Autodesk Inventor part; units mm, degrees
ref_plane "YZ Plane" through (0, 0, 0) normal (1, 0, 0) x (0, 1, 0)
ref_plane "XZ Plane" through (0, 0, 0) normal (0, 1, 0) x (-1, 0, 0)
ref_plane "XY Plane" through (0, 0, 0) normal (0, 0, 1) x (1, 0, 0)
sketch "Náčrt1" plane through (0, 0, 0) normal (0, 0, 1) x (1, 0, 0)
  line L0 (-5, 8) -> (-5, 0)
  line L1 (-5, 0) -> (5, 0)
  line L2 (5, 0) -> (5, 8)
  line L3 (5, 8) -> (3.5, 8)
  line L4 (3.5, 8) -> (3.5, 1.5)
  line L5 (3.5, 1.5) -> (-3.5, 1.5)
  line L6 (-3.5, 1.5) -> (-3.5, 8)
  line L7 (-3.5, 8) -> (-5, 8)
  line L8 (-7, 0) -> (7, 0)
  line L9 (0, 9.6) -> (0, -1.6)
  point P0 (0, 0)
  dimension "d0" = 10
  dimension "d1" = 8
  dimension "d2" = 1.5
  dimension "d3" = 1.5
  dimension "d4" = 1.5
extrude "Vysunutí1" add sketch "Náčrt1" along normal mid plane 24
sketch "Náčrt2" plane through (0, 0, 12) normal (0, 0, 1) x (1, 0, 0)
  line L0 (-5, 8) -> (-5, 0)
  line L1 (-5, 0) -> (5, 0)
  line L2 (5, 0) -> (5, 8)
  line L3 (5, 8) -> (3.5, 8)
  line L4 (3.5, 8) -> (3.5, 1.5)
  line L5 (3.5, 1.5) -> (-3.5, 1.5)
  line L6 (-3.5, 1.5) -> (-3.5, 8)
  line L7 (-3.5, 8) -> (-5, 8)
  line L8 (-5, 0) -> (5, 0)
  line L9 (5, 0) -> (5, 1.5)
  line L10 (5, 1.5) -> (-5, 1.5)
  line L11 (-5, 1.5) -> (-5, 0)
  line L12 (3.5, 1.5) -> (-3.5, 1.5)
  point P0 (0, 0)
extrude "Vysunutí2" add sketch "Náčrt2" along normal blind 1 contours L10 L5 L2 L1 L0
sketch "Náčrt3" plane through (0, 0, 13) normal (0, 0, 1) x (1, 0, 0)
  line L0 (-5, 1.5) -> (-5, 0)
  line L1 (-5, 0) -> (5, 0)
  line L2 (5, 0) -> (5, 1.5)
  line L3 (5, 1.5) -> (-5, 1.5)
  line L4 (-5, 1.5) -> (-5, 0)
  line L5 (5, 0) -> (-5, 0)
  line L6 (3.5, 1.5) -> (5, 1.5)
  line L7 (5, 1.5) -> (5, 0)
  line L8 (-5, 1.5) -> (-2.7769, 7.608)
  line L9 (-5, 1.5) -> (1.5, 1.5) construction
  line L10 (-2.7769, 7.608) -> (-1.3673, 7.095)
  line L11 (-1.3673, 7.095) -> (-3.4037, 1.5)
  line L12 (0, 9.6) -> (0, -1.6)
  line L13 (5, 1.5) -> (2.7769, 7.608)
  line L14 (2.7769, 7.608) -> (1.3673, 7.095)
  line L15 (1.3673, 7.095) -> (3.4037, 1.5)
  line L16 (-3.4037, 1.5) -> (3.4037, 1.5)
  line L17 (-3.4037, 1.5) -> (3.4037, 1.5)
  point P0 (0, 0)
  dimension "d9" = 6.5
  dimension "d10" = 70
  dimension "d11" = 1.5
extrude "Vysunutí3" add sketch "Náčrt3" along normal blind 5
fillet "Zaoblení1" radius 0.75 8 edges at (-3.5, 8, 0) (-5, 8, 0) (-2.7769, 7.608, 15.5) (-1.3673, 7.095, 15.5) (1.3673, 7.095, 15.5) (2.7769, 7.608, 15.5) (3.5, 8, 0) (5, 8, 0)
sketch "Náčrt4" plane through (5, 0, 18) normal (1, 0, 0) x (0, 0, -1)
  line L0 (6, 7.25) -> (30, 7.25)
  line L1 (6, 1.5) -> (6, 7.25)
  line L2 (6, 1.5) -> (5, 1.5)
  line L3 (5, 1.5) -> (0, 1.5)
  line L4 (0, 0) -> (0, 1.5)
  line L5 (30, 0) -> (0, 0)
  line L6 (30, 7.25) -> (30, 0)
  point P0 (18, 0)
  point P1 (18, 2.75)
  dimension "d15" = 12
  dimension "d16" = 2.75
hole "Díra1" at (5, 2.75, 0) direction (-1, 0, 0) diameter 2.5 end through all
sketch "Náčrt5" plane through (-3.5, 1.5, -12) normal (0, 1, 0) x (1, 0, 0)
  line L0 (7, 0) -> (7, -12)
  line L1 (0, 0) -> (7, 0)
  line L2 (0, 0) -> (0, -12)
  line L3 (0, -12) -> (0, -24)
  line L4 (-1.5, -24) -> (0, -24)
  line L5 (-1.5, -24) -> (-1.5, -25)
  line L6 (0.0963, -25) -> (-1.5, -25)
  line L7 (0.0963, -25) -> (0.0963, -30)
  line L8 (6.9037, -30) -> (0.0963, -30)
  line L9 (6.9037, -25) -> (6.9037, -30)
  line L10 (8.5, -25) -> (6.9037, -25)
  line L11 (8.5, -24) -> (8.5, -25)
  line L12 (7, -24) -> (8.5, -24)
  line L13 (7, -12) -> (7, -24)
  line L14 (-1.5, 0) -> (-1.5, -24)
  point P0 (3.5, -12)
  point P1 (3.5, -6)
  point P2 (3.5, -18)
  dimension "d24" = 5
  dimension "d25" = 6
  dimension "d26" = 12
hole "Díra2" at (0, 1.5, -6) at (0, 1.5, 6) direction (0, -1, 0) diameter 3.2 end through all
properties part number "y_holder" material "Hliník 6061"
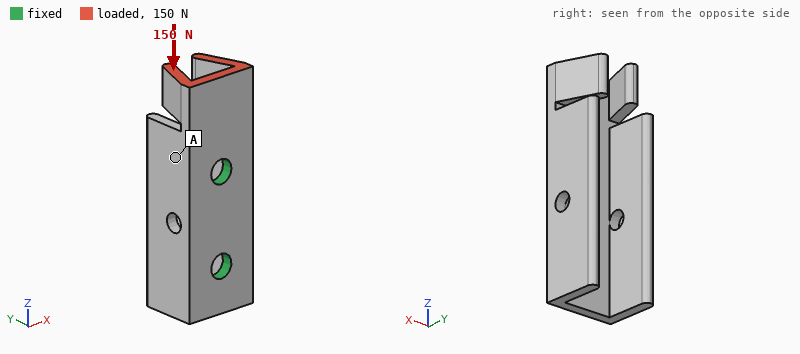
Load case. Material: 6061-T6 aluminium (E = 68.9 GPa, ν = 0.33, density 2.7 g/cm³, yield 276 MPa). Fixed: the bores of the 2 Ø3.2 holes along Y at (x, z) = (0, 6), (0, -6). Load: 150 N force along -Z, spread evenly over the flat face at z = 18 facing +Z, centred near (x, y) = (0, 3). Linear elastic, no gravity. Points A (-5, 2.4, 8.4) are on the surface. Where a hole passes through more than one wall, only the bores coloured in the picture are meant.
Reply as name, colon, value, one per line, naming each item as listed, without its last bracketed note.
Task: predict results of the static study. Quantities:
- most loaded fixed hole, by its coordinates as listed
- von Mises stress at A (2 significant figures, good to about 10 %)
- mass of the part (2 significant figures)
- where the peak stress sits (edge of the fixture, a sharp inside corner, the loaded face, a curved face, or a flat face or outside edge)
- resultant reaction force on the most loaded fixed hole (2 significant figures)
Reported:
most loaded fixed hole, by its coordinates as listed: (0, 6)
von Mises stress at A: 12 MPa
mass of the part: 2.6 g
where the peak stress sits: a flat face or outside edge
resultant reaction force on the most loaded fixed hole: 110 N
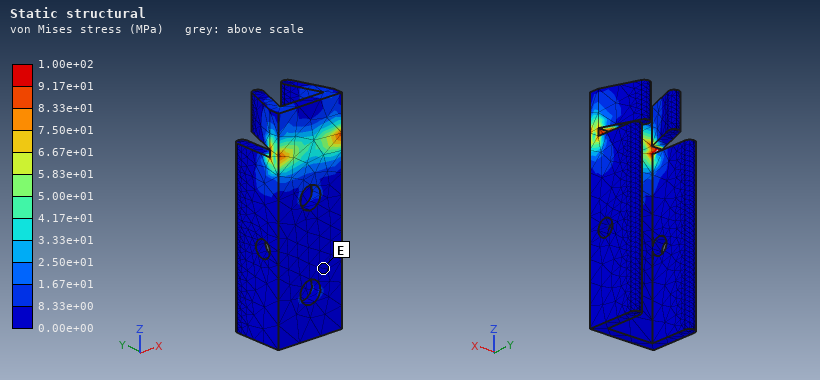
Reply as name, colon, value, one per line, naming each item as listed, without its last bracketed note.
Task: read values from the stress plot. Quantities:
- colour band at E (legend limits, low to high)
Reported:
colour band at E: 0.00e+00 to 8.33e+00 MPa
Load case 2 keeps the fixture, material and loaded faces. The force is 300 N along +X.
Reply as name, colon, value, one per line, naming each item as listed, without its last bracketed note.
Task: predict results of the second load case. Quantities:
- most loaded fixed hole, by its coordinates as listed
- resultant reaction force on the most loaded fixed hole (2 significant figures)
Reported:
most loaded fixed hole, by its coordinates as listed: (0, 6)
resultant reaction force on the most loaded fixed hole: 450 N
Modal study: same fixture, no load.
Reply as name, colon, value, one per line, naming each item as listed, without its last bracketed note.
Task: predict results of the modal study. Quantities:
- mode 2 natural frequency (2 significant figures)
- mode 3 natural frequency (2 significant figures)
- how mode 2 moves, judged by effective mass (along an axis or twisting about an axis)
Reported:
mode 2 natural frequency: 12 kHz
mode 3 natural frequency: 15 kHz
how mode 2 moves, judged by effective mass: along X
